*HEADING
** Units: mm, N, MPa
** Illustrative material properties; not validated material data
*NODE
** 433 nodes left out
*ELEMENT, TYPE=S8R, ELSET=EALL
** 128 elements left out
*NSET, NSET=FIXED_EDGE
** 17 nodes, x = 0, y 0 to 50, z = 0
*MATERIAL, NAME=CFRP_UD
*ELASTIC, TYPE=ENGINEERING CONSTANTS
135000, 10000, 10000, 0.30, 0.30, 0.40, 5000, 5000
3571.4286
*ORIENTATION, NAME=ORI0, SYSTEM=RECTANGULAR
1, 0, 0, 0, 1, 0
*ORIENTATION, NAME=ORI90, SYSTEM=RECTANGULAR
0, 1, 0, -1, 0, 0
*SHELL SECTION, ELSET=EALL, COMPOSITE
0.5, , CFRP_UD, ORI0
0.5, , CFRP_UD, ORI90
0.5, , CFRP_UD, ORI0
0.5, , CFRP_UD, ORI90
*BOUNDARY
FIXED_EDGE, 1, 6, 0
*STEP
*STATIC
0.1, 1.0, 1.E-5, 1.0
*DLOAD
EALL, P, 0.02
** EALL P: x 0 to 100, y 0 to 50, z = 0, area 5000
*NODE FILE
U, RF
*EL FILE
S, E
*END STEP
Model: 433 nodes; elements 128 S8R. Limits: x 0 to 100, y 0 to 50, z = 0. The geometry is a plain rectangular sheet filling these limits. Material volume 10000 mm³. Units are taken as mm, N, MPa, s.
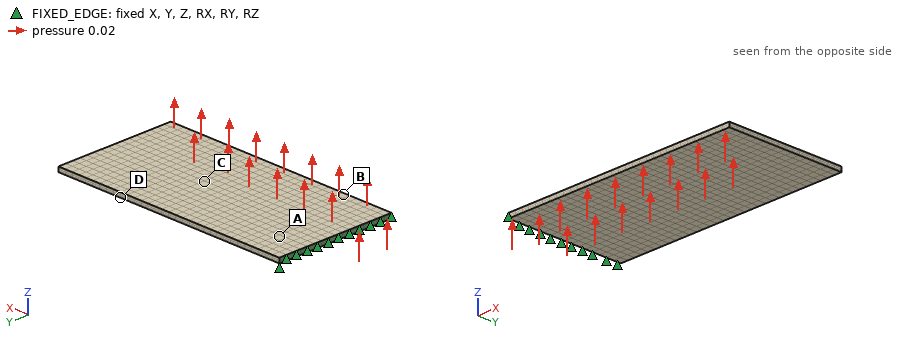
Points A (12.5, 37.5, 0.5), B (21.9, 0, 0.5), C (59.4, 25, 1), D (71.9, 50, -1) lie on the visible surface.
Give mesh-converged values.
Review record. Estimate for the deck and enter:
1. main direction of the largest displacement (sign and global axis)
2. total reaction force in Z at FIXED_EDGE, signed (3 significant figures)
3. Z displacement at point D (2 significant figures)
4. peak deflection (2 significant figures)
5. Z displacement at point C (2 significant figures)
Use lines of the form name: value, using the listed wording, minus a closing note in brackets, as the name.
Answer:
main direction of the largest displacement: +Z
total reaction force in Z at FIXED_EDGE, signed: -100 N
Z displacement at point D: 3.8 mm
peak deflection: 6.0 mm
Z displacement at point C: 2.8 mm
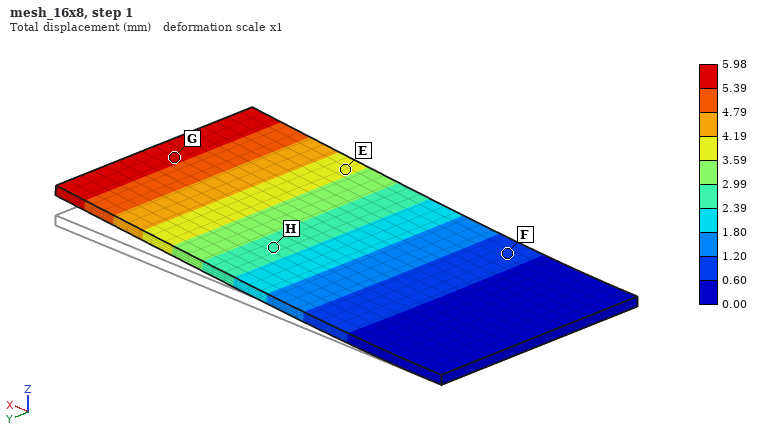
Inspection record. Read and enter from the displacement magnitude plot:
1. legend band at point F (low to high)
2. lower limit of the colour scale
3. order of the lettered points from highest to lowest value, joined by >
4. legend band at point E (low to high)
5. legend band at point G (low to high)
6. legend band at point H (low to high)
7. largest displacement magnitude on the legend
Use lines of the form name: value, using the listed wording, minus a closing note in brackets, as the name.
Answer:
legend band at point F: 0.60 to 1.20 mm
lower limit of the colour scale: 0.00 mm
order of the lettered points from highest to lowest value, joined by >: G > E > H > F
legend band at point E: 3.59 to 4.19 mm
legend band at point G: 5.39 to 5.98 mm
legend band at point H: 2.39 to 2.99 mm
largest displacement magnitude on the legend: 5.98 mm
